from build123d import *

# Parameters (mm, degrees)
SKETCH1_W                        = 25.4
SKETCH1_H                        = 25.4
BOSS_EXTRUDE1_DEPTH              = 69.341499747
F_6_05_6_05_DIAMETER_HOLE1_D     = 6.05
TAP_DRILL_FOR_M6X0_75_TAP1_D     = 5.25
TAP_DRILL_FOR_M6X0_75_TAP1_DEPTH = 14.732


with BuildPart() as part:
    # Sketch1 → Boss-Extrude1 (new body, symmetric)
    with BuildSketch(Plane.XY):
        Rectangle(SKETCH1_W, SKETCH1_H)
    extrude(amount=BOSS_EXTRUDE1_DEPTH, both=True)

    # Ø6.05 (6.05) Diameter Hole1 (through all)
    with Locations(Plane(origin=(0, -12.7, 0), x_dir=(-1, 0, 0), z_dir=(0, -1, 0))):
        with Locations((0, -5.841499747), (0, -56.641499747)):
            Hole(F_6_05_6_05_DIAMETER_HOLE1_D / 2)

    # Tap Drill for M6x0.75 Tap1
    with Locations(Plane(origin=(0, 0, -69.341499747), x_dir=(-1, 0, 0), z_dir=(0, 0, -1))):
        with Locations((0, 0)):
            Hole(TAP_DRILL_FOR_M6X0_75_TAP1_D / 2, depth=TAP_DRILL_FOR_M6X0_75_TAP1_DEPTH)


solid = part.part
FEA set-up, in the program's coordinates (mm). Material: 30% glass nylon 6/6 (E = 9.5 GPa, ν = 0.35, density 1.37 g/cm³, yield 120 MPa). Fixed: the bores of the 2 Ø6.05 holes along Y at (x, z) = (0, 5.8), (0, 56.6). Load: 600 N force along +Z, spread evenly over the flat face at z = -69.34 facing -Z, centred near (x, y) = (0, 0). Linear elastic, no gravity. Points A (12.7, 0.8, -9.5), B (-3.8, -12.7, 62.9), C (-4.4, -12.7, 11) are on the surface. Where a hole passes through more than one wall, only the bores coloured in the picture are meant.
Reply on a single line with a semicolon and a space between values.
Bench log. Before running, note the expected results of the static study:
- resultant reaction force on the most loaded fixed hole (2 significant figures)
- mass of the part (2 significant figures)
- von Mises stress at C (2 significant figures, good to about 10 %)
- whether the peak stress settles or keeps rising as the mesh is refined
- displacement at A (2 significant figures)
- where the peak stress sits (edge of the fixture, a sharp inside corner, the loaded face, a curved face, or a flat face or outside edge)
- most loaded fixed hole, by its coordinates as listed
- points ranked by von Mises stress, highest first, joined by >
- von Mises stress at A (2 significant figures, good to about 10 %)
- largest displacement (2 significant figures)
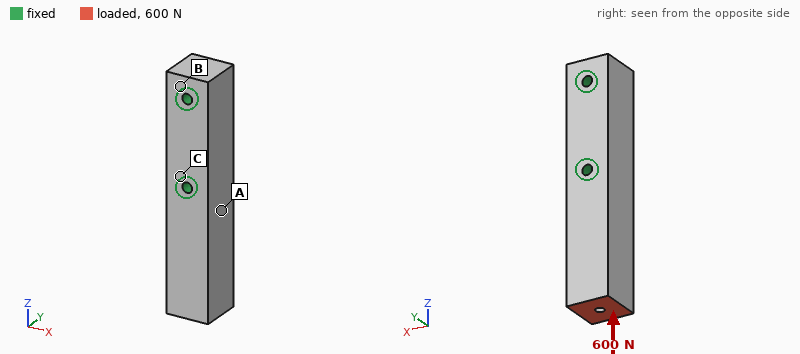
550 N; 120 g; 0.45 MPa; keeps rising; 1.9 µm; edge of the fixture; (0, 5.8); A > C > B; 0.82 MPa; 7.8 µm
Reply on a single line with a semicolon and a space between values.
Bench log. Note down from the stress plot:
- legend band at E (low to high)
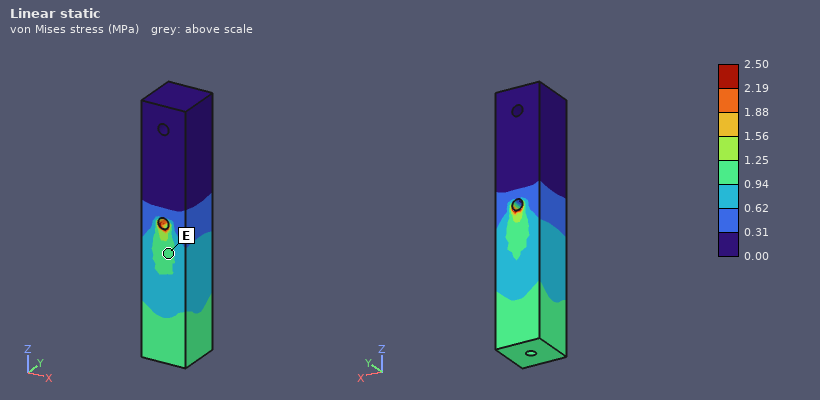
0.94 to 1.25 MPa
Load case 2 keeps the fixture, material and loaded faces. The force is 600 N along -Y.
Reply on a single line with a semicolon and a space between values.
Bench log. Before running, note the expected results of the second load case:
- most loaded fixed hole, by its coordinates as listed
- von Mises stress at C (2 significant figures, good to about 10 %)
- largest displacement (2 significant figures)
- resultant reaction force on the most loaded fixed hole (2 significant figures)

(0, 5.8); 4.5 MPa; 0.31 mm; 770 N
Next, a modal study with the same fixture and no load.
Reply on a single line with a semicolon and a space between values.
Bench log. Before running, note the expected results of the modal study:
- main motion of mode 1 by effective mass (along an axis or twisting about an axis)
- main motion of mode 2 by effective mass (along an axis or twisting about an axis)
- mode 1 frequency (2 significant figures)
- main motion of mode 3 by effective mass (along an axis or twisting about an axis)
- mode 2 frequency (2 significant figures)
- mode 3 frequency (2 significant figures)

along X; along Y; 1400 Hz; twisting about Z; 1700 Hz; 4800 Hz
